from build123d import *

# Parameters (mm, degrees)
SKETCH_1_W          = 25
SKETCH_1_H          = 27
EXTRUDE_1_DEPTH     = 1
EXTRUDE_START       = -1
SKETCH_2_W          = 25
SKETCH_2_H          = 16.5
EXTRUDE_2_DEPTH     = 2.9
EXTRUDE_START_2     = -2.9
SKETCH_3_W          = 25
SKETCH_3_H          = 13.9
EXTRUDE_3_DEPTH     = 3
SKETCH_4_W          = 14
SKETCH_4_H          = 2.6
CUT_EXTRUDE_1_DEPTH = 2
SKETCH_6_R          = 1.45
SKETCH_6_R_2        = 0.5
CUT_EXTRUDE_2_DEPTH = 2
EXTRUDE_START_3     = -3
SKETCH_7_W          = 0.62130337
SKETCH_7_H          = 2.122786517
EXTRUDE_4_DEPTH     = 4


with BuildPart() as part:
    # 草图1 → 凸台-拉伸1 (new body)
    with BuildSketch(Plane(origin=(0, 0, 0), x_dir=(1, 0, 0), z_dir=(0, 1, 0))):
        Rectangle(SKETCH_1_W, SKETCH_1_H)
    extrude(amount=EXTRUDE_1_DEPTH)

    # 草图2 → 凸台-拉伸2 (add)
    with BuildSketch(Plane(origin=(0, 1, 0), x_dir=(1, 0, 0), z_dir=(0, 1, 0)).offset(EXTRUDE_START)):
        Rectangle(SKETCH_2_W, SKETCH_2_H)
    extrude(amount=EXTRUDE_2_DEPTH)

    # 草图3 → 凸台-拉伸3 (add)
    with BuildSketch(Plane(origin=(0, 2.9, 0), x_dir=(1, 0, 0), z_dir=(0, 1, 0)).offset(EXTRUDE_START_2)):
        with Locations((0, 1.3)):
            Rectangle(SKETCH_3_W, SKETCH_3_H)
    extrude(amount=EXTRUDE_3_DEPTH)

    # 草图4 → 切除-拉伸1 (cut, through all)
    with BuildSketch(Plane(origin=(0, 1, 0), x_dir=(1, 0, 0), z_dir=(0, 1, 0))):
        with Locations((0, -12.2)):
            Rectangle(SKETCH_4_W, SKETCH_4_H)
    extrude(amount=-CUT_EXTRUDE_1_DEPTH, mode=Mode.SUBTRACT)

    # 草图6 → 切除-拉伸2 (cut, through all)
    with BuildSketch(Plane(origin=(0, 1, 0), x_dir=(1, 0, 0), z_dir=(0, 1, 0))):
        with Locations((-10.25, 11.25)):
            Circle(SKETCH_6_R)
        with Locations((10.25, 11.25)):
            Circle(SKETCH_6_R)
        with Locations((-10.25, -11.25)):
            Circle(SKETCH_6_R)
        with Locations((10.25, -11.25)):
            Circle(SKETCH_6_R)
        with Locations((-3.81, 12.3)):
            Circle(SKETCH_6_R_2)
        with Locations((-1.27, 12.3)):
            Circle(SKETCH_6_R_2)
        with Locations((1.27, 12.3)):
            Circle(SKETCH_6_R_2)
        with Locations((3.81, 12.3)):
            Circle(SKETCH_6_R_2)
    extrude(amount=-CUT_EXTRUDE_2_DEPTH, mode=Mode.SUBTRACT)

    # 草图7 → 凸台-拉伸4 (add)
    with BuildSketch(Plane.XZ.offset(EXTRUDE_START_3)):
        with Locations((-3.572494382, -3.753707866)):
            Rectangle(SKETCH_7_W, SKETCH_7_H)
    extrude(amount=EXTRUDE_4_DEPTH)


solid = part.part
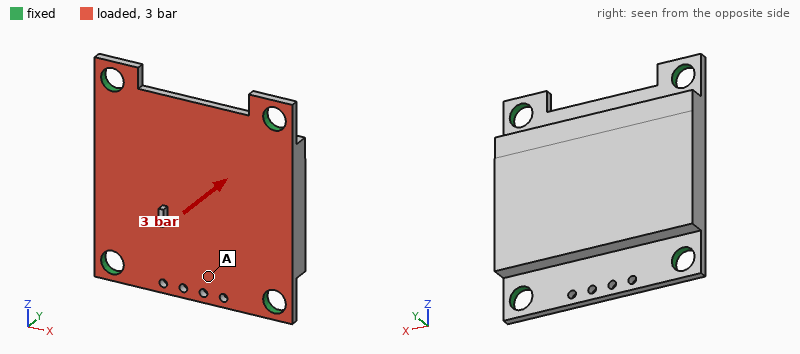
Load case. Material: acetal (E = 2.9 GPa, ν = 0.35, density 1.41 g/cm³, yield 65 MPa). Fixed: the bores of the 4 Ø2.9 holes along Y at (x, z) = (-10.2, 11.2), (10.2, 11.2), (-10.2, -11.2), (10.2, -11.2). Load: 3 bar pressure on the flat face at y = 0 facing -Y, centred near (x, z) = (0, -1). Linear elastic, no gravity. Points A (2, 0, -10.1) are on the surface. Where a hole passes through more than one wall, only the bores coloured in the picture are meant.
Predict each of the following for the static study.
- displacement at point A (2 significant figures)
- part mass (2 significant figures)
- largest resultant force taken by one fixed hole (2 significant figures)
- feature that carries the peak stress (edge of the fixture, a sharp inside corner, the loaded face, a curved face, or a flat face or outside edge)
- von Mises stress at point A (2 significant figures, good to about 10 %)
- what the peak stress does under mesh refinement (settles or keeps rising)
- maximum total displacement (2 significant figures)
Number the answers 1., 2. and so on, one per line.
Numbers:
1. 0.16 mm
2. 2.0 g
3. 65 N
4. edge of the fixture
5. 9.5 MPa
6. keeps rising
7. 0.21 mm
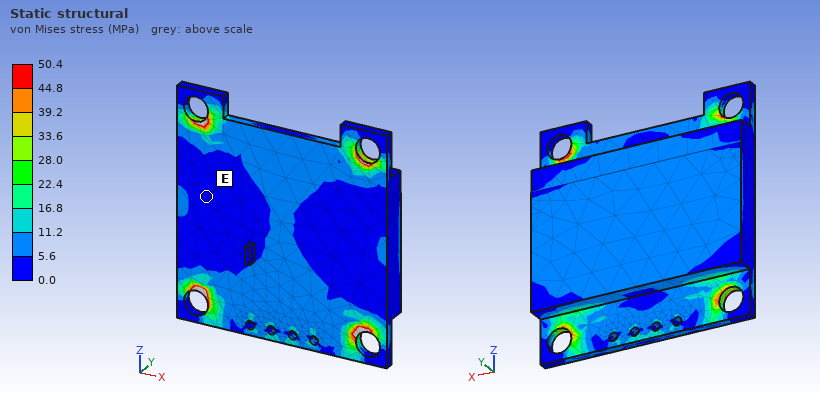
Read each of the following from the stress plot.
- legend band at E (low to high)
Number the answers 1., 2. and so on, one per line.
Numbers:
1. 0.0 to 5.6 MPa
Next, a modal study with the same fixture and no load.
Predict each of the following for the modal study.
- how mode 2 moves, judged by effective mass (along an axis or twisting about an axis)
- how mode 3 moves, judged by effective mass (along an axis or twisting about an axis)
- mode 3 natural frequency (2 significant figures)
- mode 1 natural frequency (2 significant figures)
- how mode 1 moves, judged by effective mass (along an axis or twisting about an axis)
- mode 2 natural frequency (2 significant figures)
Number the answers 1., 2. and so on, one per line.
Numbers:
1. twisting about Z
2. twisting about X
3. 7000 Hz
4. 4200 Hz
5. along Y
6. 6600 Hz
